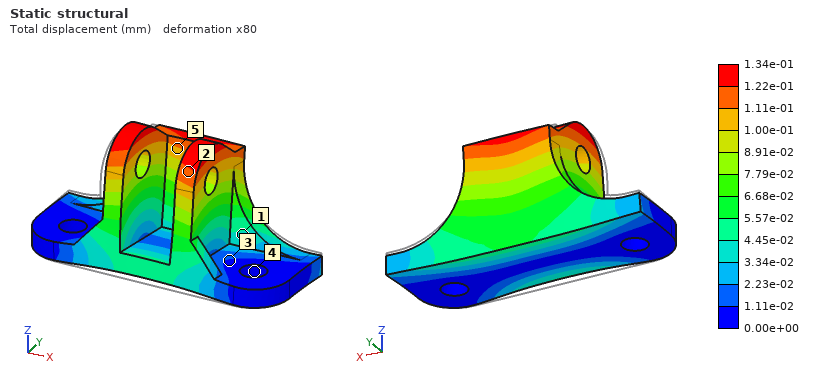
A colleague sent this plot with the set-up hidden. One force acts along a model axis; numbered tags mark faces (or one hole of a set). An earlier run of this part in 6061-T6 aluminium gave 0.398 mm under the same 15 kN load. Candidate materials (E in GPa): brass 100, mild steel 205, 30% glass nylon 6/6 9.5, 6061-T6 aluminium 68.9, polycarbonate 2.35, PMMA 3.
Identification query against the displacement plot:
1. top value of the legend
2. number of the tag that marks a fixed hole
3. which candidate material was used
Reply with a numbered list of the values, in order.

1. 1.34e-01 mm
2. 4
3. mild steel
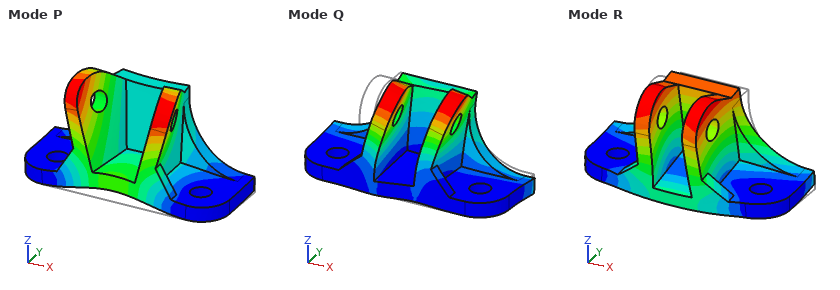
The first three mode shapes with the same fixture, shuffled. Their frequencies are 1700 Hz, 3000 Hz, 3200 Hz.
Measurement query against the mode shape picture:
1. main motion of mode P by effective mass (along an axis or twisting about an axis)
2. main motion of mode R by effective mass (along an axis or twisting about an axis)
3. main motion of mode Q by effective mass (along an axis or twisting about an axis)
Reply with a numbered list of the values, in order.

1. along Z
2. along Y
3. along X
